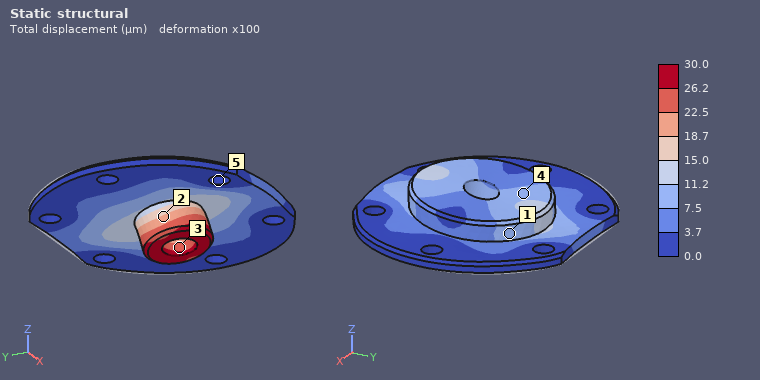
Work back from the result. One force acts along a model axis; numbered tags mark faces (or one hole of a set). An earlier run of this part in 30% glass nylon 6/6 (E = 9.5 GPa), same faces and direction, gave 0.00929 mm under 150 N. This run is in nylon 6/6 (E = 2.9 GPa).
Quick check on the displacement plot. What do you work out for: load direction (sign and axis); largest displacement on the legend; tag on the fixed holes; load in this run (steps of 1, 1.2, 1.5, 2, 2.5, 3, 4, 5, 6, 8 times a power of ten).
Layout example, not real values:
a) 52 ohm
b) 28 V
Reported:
a) -Y
b) 30.0 µm
c) 5
d) 150 N
